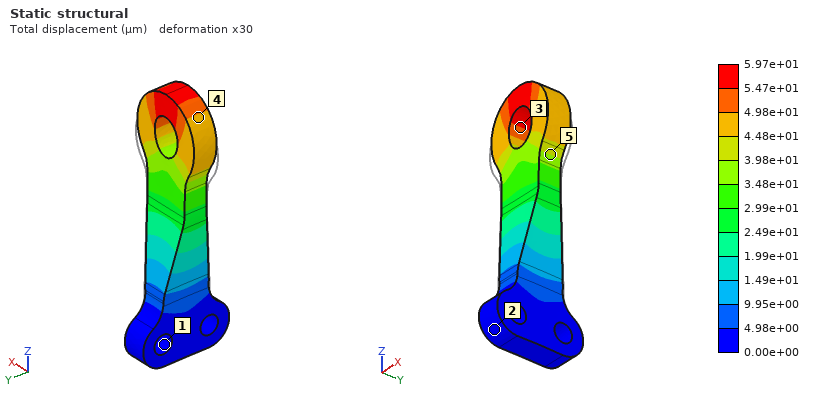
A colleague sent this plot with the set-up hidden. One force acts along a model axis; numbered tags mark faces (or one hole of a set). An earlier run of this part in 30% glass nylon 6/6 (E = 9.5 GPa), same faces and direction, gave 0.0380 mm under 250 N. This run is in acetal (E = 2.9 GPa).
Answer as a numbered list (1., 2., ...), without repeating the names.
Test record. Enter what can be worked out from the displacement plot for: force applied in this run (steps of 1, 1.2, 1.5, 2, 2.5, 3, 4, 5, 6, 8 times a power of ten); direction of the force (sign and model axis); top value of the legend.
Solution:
1. 120 N
2. +Z
3. 5.97e+01 µm
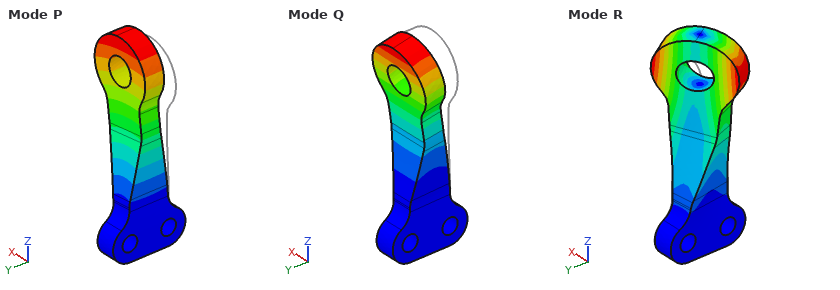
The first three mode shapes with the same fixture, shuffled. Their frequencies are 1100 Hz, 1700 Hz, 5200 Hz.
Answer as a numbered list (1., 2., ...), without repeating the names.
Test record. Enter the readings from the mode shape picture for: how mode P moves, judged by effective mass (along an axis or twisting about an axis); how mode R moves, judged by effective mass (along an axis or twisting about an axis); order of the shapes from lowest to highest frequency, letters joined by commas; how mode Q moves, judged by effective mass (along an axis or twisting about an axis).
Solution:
1. along X
2. twisting about Z
3. P, Q, R
4. along Y
